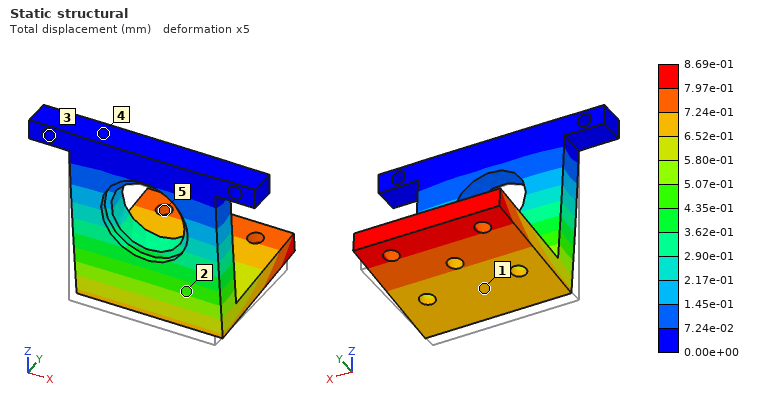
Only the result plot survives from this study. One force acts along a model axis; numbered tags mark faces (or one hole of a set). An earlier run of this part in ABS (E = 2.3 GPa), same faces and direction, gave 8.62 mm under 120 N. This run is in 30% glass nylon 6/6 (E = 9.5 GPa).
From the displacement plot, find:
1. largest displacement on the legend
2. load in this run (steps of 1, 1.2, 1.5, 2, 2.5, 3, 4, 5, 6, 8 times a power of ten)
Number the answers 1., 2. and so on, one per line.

1. 8.69e-01 mm
2. 50 N
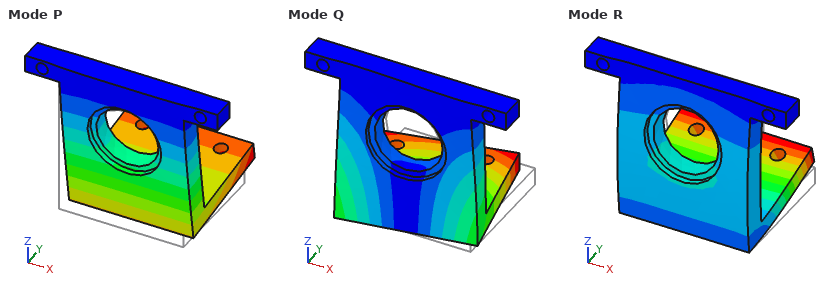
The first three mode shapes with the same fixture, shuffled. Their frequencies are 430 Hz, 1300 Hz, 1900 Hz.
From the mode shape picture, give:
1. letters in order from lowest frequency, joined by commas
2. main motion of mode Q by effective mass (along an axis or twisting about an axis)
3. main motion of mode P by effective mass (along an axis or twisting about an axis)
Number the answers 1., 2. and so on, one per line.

1. P, Q, R
2. along X
3. along Y
